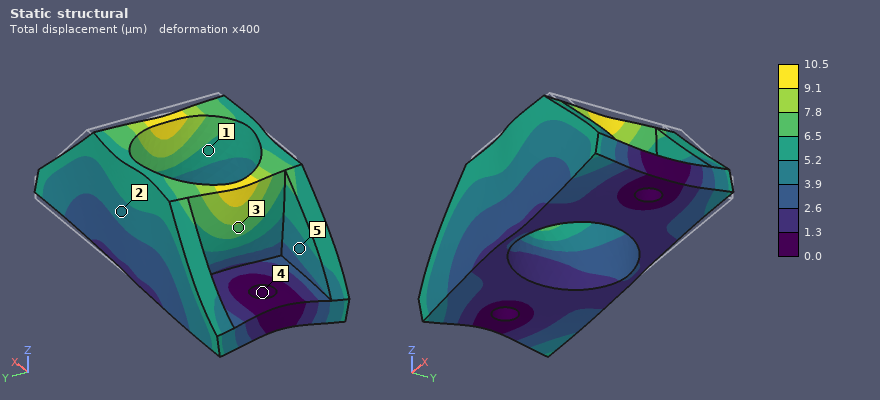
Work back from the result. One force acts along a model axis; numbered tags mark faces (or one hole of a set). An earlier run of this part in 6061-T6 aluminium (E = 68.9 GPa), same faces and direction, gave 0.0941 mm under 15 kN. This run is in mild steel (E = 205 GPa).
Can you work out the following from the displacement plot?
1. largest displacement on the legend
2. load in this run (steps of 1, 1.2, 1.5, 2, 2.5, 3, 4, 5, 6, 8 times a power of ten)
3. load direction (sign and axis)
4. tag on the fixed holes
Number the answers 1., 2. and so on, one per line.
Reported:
1. 10.5 µm
2. 5 kN
3. -X
4. 4
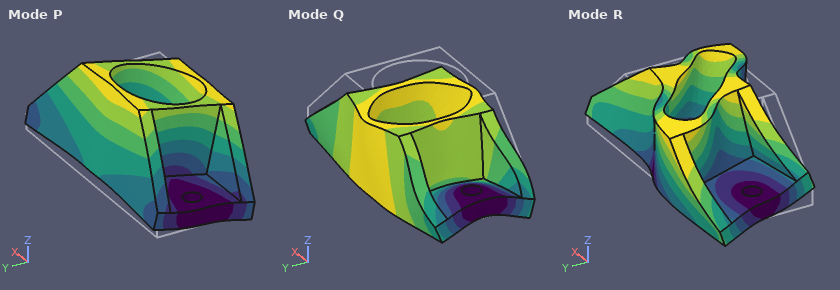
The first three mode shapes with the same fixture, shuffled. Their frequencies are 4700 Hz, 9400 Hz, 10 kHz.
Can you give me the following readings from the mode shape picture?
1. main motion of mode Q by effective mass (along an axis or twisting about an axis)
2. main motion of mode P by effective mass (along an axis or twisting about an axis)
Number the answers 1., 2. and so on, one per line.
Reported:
1. along Z
2. along Y
